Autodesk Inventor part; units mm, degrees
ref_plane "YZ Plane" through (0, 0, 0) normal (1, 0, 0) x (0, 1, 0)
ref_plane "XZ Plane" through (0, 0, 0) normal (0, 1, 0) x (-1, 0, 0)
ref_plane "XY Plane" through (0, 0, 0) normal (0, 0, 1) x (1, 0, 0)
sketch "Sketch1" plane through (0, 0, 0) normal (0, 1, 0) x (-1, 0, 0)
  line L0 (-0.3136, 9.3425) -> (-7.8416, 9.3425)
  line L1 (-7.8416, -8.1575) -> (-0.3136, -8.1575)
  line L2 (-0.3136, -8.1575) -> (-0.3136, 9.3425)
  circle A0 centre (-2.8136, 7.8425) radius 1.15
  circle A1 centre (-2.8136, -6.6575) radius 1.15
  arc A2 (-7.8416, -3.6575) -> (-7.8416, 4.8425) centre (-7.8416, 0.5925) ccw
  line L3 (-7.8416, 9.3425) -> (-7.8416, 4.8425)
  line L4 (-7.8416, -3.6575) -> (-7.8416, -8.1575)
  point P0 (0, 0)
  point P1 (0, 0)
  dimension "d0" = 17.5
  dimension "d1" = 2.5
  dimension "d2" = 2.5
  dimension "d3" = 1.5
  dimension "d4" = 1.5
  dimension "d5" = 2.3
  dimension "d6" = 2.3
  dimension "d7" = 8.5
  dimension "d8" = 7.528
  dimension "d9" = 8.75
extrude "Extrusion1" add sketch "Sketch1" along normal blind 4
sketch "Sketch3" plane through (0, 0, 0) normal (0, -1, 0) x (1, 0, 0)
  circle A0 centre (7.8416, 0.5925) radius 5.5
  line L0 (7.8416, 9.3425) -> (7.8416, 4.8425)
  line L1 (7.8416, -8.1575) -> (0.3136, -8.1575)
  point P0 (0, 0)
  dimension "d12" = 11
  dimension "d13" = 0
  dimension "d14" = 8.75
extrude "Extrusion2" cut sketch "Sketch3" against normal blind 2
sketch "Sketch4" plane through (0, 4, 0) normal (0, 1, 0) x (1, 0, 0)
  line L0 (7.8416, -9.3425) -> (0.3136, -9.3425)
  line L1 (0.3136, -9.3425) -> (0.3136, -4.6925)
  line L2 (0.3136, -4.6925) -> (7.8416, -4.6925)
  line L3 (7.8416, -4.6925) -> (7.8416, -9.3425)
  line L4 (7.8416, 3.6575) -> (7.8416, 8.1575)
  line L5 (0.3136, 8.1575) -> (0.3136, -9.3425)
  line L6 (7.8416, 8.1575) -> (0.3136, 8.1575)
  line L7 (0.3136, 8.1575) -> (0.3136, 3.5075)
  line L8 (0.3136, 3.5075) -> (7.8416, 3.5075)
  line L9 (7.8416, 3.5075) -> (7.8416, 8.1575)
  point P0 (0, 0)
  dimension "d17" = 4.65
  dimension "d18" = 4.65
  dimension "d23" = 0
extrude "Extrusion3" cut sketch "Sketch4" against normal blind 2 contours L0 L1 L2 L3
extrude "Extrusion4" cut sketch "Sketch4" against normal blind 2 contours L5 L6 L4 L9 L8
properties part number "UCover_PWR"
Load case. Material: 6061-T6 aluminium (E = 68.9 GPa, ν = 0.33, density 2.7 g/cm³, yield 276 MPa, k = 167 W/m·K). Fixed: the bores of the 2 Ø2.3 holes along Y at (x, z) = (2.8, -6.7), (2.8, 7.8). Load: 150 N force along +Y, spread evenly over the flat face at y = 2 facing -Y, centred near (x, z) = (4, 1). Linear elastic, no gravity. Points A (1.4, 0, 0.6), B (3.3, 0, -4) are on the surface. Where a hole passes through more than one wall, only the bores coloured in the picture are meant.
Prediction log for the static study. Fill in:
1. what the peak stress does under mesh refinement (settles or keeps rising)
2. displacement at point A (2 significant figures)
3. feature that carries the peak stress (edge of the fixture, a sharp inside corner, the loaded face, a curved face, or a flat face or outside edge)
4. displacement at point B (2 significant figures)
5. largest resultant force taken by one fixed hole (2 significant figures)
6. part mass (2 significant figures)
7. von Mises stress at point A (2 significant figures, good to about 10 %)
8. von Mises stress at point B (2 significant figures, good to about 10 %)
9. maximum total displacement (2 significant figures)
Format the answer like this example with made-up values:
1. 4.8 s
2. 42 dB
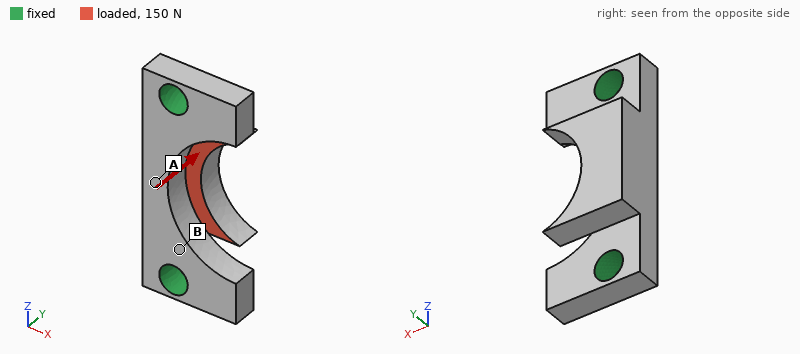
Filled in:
1. keeps rising
2. 2.6 µm
3. a sharp inside corner
4. 2.0 µm
5. 88 N
6. 0.59 g
7. 15 MPa
8. 27 MPa
9. 11 µm
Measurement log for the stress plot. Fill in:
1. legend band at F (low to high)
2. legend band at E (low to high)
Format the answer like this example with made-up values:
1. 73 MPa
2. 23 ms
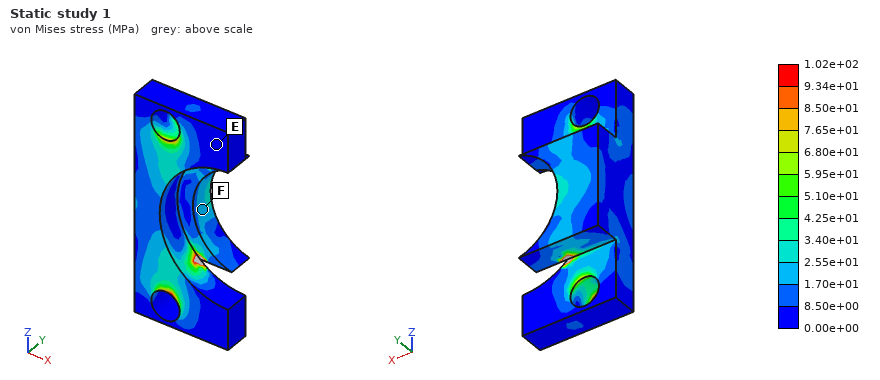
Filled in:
1. 1.70e+01 to 2.55e+01 MPa
2. 0.00e+00 to 8.50e+00 MPa
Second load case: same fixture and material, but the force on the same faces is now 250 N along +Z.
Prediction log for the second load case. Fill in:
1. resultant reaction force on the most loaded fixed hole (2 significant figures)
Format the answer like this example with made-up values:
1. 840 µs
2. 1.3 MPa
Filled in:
1. 130 N
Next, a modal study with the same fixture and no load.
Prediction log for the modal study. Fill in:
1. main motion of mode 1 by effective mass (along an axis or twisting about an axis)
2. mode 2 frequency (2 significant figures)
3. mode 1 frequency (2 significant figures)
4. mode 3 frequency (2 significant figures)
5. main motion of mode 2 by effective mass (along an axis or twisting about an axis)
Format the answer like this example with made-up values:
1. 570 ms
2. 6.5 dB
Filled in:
1. along X
2. 63 kHz
3. 47 kHz
4. 83 kHz
5. along Y
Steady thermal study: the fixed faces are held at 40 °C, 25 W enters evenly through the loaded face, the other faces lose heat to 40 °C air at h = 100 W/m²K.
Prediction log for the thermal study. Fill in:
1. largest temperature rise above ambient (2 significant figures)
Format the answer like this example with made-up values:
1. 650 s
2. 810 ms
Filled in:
1. 61 K
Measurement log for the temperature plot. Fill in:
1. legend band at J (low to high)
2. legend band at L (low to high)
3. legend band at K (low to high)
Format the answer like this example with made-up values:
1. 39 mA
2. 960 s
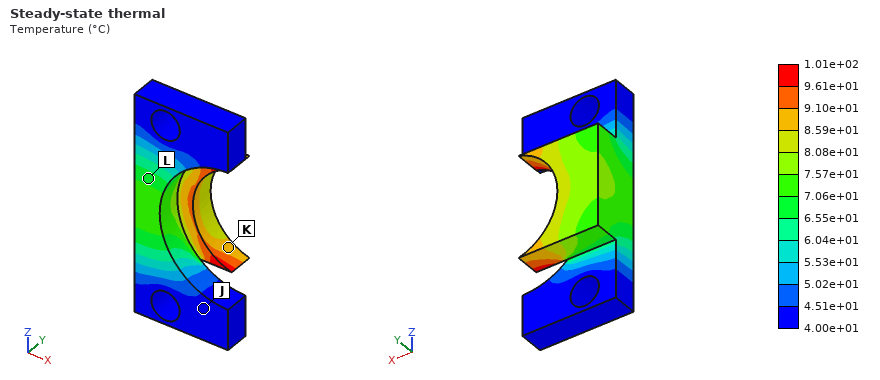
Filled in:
1. 4.00e+01 to 4.51e+01 °C
2. 6.55e+01 to 7.06e+01 °C
3. 8.59e+01 to 9.10e+01 °C
